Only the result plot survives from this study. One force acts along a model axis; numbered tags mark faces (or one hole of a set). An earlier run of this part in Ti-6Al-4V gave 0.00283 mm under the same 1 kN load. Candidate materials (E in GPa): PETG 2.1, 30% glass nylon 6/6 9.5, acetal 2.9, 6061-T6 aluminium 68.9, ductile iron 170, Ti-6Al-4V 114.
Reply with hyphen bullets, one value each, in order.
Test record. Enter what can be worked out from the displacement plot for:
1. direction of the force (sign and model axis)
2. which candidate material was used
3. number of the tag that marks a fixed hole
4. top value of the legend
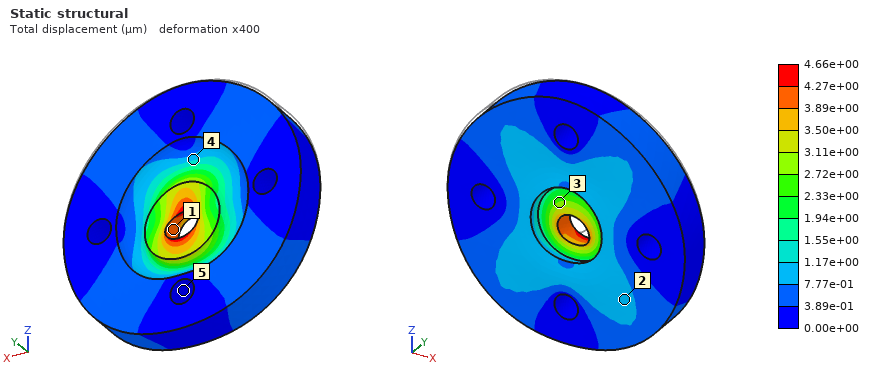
- -Z
- 6061-T6 aluminium
- 5
- 4.66e+00 µm
